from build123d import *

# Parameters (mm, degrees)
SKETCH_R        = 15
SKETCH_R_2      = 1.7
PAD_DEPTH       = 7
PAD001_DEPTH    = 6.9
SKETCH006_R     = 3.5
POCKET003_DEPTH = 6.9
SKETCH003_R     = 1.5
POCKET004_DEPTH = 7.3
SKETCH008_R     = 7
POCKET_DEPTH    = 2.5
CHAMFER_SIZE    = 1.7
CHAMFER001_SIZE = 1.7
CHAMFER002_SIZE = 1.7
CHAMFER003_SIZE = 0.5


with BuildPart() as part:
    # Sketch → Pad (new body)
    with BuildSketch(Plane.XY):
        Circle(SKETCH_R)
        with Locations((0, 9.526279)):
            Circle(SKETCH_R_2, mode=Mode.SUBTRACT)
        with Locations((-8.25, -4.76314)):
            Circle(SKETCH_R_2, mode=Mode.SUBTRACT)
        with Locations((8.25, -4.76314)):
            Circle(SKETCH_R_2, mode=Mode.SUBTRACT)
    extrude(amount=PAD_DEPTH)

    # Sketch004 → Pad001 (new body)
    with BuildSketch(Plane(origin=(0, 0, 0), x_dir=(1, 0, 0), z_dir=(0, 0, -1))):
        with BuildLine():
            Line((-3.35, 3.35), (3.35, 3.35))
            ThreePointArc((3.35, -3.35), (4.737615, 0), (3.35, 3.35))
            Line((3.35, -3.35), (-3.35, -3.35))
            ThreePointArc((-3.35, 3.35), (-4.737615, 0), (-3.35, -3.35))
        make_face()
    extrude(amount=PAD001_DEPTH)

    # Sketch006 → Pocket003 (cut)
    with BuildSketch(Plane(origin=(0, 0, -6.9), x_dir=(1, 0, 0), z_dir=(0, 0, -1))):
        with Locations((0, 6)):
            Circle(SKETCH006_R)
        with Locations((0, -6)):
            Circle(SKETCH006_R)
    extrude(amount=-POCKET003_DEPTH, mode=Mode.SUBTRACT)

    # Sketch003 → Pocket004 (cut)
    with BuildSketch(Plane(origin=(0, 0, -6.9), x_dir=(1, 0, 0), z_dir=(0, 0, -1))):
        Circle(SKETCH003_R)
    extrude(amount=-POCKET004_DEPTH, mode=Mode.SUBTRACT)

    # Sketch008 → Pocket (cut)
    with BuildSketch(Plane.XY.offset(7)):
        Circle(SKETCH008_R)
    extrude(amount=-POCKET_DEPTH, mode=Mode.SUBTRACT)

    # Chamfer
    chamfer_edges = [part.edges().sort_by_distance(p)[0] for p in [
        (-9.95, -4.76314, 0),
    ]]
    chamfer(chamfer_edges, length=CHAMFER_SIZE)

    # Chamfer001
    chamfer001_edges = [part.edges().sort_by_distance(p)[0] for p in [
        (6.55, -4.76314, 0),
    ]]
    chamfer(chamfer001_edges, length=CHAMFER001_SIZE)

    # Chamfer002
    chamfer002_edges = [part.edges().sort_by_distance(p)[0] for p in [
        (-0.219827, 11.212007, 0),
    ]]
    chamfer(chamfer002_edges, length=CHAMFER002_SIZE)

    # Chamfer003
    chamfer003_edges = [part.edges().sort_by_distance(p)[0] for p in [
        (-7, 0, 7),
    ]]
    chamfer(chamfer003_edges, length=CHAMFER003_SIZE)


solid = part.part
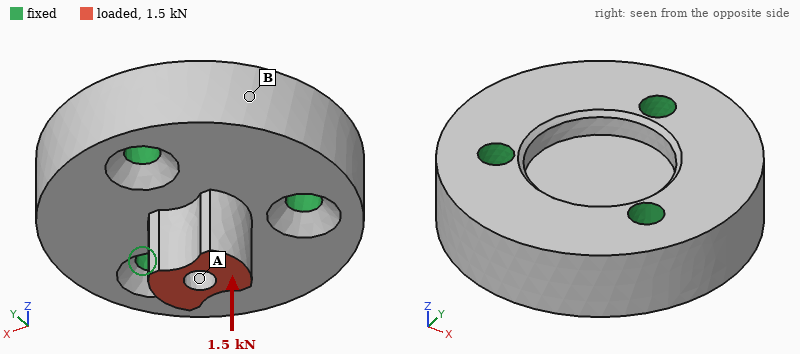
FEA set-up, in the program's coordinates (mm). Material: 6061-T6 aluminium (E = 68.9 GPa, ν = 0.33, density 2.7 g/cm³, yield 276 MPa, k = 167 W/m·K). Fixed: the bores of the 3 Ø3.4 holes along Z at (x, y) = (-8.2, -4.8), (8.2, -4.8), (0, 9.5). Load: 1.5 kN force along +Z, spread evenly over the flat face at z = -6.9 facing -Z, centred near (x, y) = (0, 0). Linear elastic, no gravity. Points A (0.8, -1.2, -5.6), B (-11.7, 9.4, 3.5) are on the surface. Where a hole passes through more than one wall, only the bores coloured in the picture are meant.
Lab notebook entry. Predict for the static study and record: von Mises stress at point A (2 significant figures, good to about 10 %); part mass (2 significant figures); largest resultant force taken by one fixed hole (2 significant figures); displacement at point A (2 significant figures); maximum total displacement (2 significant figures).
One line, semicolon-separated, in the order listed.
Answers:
33 MPa; 12 g; 560 N; 6.4 µm; 7.6 µm
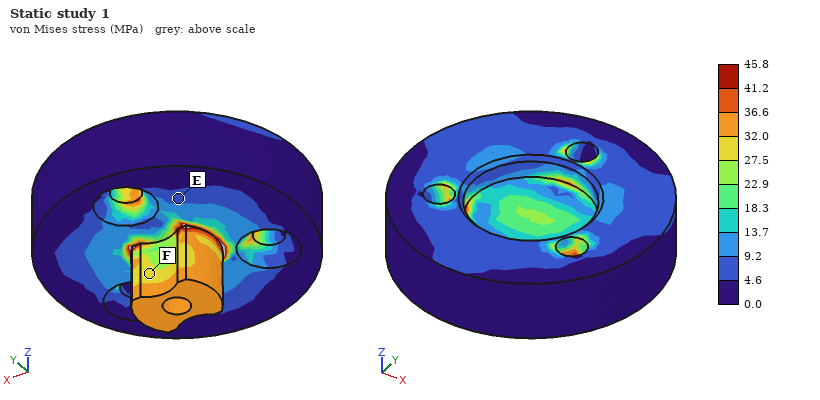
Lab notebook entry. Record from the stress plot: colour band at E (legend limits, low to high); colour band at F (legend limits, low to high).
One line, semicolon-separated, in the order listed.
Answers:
4.6 to 9.2 MPa; 27.5 to 32.0 MPa
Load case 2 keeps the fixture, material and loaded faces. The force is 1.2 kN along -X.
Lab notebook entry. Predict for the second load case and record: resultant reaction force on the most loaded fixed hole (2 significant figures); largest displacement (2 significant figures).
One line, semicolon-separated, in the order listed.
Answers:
850 N; 32 µm
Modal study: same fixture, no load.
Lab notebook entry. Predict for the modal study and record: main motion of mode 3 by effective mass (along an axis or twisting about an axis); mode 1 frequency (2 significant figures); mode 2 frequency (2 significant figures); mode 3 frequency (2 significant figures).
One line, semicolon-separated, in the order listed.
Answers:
along Z; 37 kHz; 38 kHz; 43 kHz
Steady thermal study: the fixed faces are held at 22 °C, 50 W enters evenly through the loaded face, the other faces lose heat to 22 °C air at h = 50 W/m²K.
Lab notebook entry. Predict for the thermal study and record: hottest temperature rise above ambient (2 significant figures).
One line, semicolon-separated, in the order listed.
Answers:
63 K
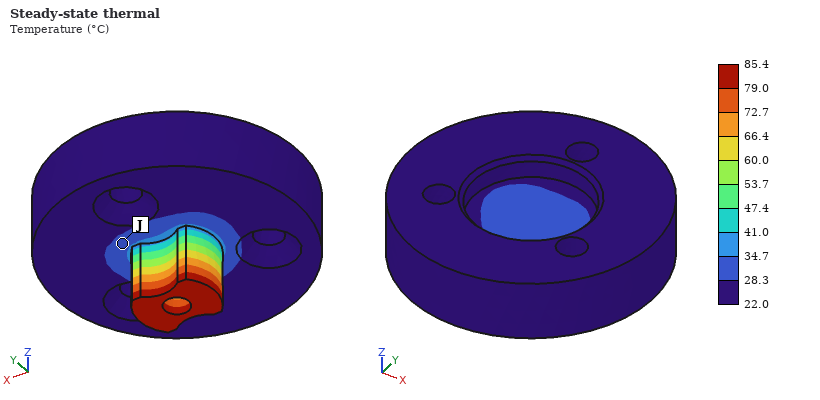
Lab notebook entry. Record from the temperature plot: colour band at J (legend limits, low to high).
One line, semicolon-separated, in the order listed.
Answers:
28.3 to 34.7 °C
